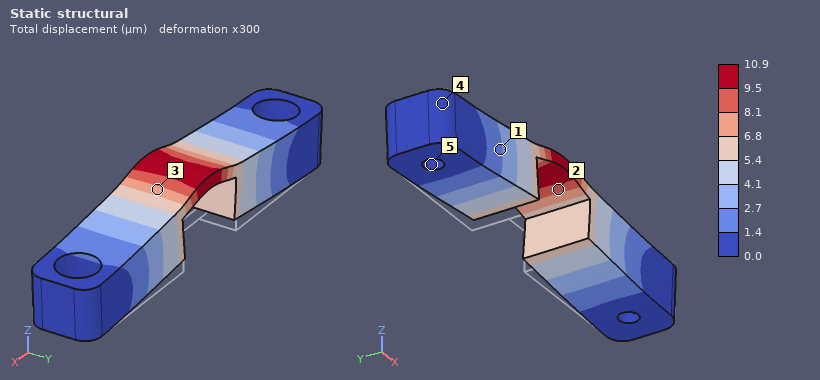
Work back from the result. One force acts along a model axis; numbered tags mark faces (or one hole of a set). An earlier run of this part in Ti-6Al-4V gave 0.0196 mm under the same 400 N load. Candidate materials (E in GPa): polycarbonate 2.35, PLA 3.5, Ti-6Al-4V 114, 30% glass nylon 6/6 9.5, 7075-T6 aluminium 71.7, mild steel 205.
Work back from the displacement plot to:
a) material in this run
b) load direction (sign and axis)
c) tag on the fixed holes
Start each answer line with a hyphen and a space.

- mild steel
- +Z
- 5
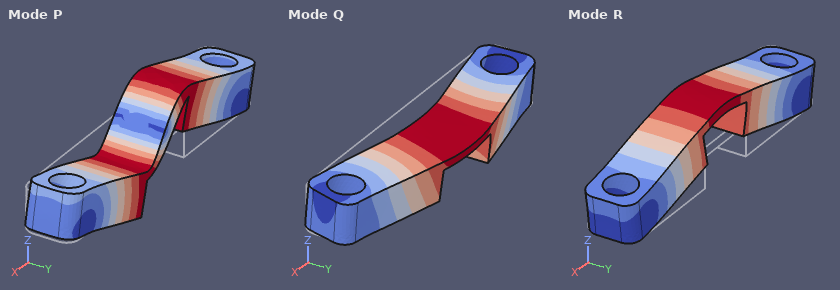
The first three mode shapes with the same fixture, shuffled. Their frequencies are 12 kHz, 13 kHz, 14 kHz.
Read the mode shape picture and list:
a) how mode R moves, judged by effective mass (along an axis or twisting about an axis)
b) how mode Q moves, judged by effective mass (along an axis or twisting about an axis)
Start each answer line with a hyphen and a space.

- along Z
- along Y
